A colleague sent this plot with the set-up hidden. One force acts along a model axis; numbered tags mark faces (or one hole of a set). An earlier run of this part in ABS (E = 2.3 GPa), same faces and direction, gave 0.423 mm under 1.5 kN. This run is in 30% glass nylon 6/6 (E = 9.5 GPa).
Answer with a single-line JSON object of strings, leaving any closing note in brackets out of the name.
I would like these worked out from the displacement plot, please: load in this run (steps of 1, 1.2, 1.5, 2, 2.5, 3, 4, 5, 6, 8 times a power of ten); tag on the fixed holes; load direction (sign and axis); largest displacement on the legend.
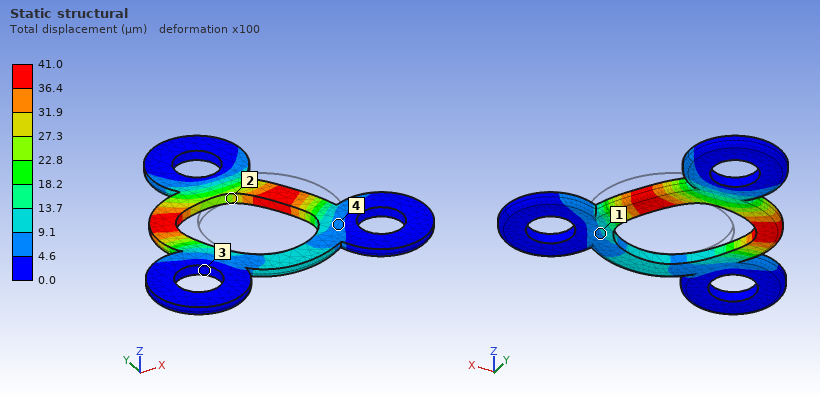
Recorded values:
{"load in this run": "600 N", "tag on the fixed holes": "3", "load direction": "-X", "largest displacement on the legend": "41.0 µm"}
